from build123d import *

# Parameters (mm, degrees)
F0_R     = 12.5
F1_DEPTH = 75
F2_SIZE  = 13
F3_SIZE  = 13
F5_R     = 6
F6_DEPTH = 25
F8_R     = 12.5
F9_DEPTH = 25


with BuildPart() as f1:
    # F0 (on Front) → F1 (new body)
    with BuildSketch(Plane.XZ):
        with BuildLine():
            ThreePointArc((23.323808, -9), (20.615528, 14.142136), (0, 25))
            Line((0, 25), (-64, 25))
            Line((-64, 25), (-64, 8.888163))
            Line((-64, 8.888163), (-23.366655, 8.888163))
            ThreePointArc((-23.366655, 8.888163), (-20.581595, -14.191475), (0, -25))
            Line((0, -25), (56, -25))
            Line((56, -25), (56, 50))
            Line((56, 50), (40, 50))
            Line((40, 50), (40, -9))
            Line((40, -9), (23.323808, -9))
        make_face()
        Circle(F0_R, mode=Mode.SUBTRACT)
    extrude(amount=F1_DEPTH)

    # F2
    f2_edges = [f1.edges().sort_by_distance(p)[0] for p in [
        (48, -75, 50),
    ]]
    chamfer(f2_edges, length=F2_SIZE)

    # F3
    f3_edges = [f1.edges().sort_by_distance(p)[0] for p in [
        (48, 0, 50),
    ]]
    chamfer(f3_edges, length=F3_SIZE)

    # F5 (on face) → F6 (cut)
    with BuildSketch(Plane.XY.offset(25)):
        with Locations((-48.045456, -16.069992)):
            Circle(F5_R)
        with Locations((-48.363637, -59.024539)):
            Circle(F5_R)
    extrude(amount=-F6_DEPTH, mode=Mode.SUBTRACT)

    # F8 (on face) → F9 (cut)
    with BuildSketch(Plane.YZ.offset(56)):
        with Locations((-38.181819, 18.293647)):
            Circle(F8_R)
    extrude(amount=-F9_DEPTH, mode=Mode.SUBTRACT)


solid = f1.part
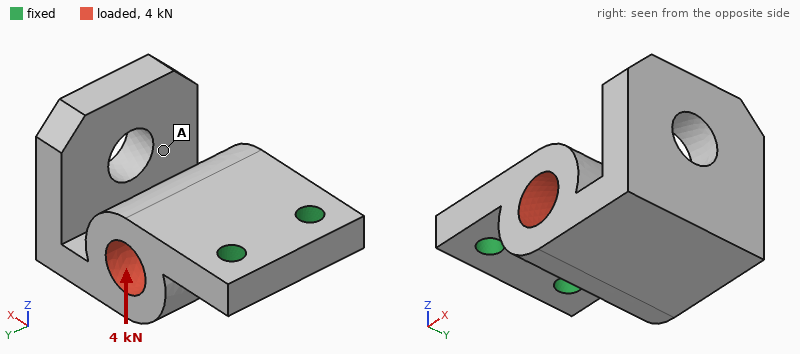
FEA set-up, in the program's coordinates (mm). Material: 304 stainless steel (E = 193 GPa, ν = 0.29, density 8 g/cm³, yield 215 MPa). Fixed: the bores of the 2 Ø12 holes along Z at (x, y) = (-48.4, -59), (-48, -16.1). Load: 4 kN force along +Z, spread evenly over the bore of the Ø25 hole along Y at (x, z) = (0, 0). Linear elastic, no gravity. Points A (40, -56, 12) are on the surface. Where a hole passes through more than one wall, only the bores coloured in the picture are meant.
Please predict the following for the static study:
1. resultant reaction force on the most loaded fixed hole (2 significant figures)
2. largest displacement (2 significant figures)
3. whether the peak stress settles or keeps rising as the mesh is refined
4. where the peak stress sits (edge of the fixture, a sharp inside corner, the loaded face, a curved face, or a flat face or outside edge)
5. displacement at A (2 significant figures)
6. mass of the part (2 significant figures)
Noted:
2.0 kN
80 µm
keeps rising
edge of the fixture
61 µm
2.2 kg
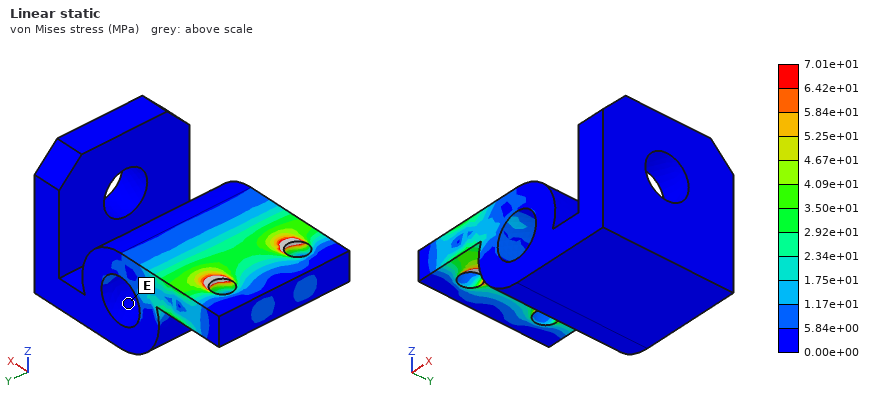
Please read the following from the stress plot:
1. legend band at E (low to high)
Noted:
0.00e+00 to 5.84e+00 MPa
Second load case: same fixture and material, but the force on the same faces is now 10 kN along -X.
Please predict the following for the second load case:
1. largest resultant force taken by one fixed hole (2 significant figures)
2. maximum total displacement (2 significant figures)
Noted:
5.1 kN
0.10 mm
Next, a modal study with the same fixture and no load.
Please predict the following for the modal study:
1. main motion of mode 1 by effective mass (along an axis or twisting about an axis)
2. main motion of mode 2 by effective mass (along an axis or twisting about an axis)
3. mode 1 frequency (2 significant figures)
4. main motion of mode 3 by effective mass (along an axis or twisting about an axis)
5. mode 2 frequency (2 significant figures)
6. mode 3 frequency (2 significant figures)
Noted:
along Z
along X
730 Hz
along Y
1800 Hz
2000 Hz
